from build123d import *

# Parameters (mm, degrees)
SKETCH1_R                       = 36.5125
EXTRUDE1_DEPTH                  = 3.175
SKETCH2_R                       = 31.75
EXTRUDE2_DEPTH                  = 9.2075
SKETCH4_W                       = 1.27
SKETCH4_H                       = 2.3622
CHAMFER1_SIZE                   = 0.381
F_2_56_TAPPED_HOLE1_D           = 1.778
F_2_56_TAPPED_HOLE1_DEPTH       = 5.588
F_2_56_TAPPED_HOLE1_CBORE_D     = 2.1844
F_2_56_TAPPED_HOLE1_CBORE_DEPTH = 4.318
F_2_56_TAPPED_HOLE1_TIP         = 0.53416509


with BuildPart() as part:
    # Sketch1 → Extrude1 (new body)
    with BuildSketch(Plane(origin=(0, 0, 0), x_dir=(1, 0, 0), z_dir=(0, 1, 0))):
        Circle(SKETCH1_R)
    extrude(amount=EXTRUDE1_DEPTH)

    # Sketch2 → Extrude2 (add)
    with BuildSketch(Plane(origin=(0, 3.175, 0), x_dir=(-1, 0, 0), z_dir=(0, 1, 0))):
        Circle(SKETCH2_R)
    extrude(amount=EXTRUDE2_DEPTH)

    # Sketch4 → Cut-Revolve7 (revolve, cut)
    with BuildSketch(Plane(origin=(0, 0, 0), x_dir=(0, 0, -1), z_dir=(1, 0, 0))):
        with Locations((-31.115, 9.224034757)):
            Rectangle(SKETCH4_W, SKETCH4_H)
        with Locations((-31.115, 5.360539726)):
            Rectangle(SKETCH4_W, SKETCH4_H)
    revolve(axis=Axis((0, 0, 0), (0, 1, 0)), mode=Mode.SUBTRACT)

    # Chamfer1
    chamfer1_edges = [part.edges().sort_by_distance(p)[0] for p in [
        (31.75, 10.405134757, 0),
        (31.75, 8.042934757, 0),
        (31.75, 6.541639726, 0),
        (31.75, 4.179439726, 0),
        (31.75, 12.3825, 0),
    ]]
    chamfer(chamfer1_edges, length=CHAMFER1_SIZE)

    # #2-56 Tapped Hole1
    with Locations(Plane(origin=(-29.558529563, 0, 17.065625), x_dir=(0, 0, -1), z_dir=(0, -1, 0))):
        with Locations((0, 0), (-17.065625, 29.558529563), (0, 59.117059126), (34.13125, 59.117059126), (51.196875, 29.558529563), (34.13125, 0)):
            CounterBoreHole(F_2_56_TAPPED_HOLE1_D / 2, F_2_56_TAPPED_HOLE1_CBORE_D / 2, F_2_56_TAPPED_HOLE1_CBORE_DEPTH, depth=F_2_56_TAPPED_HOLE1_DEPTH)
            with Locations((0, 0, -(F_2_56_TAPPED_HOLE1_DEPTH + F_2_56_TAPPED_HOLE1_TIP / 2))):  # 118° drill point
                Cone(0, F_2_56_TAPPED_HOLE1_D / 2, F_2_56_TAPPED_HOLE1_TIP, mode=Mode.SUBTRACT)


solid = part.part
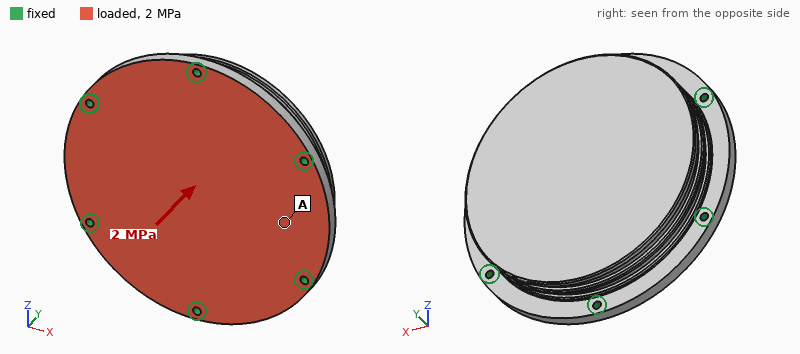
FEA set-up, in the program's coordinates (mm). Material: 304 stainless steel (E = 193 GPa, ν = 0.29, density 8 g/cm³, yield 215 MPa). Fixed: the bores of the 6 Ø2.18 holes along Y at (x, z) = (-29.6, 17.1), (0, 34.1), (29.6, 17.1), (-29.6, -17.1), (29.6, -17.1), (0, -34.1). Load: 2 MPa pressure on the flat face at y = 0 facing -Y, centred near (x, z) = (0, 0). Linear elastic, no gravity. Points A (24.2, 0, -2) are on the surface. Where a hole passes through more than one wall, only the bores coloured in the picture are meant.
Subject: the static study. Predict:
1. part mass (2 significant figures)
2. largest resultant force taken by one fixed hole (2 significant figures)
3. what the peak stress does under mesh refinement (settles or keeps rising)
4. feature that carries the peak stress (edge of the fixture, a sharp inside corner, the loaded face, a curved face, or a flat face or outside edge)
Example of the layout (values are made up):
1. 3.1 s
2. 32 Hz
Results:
1. 330 g
2. 1.6 kN
3. keeps rising
4. edge of the fixture
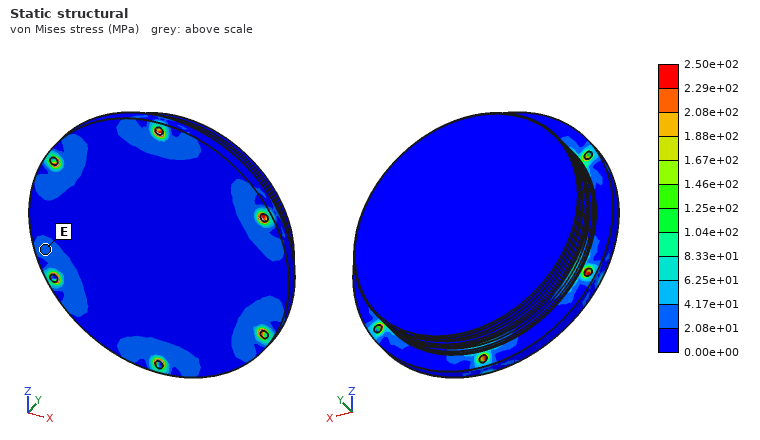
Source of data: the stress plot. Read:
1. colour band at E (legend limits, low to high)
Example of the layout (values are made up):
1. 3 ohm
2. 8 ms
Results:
1. 2.08e+01 to 4.17e+01 MPa
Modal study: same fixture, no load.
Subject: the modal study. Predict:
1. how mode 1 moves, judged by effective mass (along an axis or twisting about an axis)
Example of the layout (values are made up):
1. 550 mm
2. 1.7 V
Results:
1. along Y
